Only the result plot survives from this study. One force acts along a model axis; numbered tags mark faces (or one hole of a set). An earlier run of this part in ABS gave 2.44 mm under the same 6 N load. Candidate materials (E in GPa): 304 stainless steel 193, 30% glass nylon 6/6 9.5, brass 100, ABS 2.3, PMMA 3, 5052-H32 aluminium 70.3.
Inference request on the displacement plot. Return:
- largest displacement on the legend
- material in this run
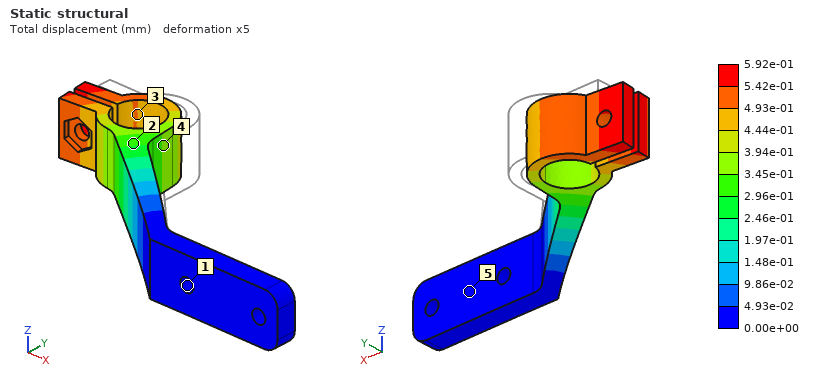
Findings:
5.92e-01 mm
30% glass nylon 6/6
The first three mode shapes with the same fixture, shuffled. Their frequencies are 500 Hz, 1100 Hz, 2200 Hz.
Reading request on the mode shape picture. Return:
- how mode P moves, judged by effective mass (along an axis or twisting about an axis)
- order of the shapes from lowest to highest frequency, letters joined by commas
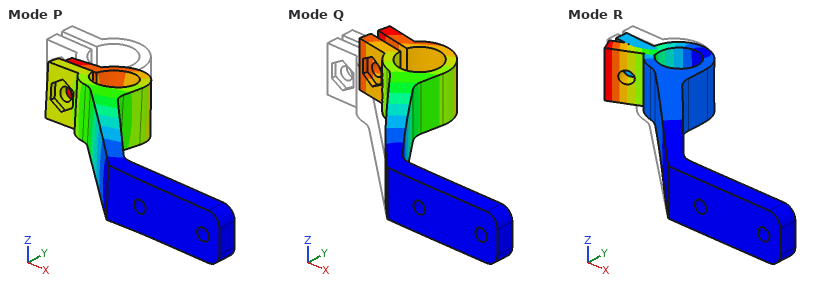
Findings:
along Z
Q, P, R
